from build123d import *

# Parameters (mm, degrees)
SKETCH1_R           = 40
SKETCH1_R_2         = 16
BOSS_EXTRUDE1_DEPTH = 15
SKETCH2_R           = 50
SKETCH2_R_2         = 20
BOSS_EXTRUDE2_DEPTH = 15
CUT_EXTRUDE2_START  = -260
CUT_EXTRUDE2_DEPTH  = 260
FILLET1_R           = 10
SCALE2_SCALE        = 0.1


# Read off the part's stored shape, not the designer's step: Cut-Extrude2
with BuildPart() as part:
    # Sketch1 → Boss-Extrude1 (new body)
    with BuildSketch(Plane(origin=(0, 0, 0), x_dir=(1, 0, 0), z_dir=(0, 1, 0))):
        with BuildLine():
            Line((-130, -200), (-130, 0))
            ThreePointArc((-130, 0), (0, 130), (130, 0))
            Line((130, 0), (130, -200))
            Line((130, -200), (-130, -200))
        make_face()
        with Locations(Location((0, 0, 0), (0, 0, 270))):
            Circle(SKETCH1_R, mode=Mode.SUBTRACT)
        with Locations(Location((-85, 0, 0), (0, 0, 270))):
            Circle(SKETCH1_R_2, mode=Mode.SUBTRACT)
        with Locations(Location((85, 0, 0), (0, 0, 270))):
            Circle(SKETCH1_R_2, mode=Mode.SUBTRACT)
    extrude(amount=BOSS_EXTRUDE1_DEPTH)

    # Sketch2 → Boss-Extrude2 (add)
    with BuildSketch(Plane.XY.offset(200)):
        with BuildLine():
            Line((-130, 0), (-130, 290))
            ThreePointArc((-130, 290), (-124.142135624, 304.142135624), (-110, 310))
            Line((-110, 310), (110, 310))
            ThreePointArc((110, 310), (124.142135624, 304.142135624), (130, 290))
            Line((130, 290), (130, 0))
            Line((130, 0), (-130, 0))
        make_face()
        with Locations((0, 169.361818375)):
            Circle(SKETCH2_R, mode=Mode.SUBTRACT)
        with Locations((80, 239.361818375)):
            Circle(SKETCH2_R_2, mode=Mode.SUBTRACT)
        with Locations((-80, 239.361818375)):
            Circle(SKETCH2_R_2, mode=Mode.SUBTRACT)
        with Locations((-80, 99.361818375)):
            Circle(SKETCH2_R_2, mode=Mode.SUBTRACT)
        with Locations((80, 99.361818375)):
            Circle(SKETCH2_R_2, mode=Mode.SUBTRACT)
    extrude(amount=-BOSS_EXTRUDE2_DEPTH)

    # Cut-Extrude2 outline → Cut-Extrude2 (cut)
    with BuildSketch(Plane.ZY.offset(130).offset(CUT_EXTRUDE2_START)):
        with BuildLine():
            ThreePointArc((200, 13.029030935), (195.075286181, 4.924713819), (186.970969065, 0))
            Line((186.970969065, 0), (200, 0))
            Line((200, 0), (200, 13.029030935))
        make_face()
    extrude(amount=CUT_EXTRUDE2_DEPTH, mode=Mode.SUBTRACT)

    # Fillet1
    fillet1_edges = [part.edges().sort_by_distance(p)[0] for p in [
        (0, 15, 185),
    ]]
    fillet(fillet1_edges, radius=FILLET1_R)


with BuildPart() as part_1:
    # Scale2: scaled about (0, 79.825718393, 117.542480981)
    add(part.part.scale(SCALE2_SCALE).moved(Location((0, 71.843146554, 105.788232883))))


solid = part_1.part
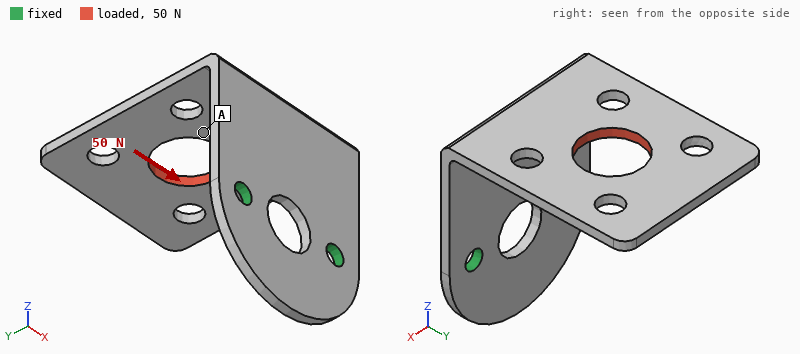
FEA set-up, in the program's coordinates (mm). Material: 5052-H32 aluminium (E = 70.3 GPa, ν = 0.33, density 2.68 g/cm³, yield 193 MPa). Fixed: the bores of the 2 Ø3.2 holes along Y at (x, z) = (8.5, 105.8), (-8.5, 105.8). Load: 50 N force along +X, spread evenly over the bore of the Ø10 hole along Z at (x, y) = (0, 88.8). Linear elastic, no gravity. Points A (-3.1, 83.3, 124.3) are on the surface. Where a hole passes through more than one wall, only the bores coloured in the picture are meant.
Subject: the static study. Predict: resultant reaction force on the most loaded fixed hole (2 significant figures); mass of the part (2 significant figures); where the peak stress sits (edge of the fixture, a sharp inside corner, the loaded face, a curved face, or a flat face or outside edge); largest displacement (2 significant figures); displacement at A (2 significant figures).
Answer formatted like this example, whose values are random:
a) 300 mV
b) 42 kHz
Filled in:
a) 68 N
b) 5.4 g
c) a flat face or outside edge
d) 0.34 mm
e) 0.12 mm
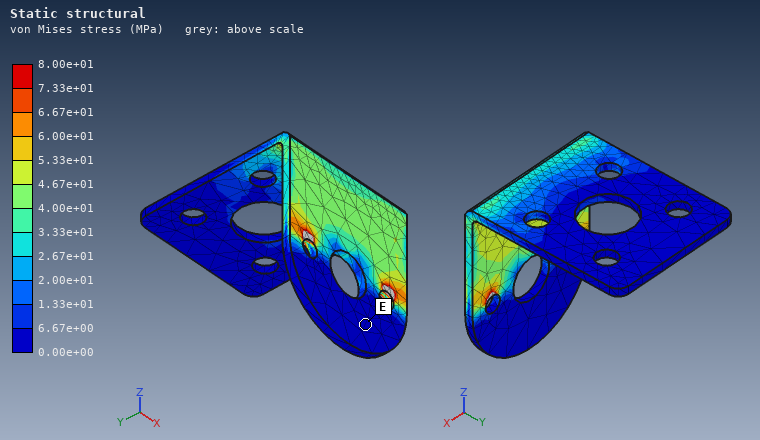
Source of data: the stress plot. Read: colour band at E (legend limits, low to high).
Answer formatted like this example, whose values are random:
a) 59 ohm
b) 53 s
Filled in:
a) 0.00e+00 to 6.67e+00 MPa
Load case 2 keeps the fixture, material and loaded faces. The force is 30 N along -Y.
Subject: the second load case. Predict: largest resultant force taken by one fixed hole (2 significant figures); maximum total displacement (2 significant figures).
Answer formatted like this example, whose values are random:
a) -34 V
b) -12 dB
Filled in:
a) 15 N
b) 0.35 mm
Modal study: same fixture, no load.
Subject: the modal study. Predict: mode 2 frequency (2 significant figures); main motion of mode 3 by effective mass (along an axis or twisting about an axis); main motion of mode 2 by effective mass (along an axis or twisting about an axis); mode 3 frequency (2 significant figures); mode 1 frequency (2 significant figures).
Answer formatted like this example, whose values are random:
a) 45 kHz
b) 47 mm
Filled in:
a) 1400 Hz
b) along Y
c) along X
d) 2100 Hz
e) 710 Hz
